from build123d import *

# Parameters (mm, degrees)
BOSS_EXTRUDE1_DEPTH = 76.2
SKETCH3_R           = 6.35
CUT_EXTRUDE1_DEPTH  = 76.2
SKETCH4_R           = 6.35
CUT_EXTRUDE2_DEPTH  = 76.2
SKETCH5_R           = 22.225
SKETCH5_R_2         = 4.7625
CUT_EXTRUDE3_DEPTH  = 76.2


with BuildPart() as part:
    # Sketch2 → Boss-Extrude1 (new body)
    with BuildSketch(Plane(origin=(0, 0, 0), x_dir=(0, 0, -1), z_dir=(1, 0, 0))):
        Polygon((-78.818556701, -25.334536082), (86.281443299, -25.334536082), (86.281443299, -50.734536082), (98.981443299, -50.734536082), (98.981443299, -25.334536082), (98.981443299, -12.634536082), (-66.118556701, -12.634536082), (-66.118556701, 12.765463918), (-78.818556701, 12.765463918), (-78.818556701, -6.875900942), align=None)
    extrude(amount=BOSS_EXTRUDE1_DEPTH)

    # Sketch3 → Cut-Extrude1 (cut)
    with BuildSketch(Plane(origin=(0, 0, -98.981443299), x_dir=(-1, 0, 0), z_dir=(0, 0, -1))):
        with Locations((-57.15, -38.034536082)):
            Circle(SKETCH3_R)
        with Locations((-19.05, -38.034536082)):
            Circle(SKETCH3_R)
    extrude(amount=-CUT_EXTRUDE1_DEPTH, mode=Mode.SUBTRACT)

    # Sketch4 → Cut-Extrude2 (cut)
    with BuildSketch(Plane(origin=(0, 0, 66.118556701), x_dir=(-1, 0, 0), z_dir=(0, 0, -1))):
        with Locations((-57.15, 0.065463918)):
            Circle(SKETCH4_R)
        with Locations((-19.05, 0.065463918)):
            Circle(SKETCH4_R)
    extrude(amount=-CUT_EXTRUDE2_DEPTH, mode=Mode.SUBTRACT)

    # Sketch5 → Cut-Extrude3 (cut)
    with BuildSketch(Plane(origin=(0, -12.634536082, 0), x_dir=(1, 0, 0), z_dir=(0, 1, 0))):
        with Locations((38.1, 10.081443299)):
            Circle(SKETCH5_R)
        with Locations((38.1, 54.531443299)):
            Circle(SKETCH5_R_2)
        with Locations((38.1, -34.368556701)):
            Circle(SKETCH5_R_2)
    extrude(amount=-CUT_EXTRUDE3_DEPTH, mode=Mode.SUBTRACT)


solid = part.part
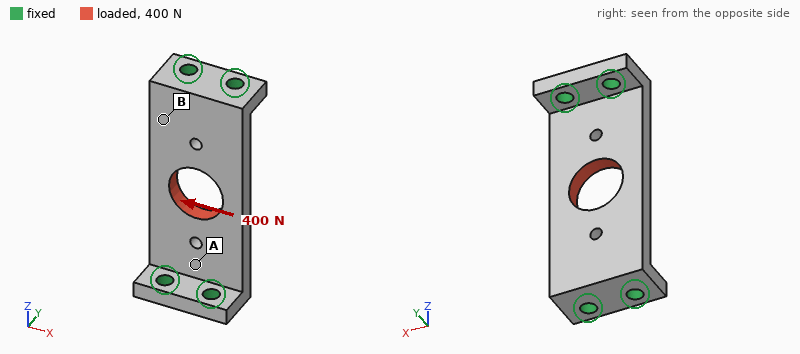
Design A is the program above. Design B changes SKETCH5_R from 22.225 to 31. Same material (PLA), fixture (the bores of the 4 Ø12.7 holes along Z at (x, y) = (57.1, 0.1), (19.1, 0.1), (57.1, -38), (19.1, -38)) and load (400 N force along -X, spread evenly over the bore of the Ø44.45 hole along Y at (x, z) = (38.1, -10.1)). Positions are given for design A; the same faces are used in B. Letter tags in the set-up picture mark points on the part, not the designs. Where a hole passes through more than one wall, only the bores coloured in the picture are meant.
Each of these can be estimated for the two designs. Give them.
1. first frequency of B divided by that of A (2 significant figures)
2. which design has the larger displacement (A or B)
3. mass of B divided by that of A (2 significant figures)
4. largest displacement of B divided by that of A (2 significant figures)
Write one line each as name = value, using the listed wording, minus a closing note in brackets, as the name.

first frequency of B divided by that of A = 1.1
which design has the larger displacement = B
mass of B divided by that of A = 0.90
largest displacement of B divided by that of A = 1.2
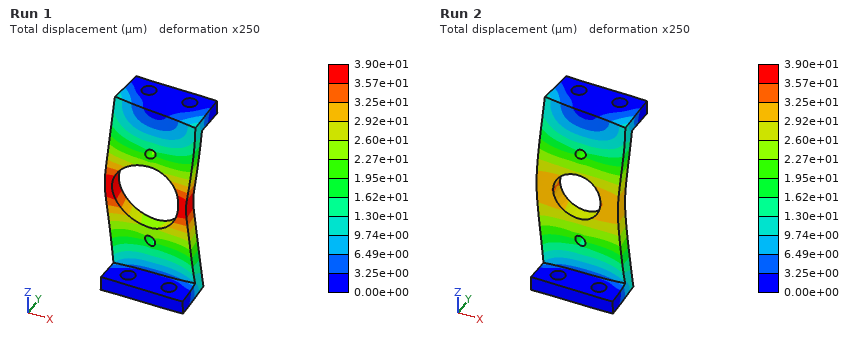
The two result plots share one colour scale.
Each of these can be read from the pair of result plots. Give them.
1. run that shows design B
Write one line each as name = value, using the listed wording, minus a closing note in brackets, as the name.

run that shows design B = Run 1
